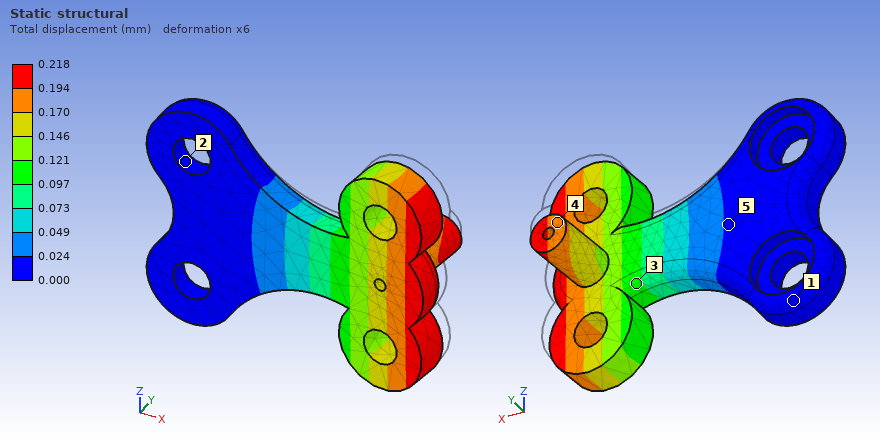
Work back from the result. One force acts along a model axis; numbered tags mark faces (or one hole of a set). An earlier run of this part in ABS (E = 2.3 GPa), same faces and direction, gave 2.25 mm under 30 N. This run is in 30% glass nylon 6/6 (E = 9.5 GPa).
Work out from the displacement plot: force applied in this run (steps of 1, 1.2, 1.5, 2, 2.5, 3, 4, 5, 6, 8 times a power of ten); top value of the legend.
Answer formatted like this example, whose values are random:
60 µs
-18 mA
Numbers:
12 N
0.218 mm
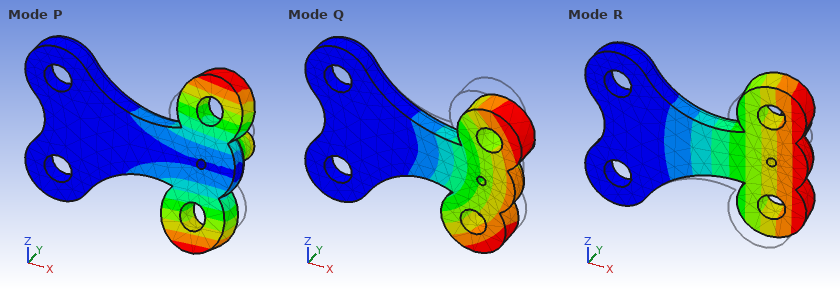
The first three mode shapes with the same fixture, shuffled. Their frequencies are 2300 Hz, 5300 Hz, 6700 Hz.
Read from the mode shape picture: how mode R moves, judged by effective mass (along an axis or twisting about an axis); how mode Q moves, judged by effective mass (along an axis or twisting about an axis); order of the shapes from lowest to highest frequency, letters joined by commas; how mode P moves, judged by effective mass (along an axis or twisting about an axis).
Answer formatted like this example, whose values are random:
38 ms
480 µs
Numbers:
along Y
along Z
R, P, Q
twisting about X
